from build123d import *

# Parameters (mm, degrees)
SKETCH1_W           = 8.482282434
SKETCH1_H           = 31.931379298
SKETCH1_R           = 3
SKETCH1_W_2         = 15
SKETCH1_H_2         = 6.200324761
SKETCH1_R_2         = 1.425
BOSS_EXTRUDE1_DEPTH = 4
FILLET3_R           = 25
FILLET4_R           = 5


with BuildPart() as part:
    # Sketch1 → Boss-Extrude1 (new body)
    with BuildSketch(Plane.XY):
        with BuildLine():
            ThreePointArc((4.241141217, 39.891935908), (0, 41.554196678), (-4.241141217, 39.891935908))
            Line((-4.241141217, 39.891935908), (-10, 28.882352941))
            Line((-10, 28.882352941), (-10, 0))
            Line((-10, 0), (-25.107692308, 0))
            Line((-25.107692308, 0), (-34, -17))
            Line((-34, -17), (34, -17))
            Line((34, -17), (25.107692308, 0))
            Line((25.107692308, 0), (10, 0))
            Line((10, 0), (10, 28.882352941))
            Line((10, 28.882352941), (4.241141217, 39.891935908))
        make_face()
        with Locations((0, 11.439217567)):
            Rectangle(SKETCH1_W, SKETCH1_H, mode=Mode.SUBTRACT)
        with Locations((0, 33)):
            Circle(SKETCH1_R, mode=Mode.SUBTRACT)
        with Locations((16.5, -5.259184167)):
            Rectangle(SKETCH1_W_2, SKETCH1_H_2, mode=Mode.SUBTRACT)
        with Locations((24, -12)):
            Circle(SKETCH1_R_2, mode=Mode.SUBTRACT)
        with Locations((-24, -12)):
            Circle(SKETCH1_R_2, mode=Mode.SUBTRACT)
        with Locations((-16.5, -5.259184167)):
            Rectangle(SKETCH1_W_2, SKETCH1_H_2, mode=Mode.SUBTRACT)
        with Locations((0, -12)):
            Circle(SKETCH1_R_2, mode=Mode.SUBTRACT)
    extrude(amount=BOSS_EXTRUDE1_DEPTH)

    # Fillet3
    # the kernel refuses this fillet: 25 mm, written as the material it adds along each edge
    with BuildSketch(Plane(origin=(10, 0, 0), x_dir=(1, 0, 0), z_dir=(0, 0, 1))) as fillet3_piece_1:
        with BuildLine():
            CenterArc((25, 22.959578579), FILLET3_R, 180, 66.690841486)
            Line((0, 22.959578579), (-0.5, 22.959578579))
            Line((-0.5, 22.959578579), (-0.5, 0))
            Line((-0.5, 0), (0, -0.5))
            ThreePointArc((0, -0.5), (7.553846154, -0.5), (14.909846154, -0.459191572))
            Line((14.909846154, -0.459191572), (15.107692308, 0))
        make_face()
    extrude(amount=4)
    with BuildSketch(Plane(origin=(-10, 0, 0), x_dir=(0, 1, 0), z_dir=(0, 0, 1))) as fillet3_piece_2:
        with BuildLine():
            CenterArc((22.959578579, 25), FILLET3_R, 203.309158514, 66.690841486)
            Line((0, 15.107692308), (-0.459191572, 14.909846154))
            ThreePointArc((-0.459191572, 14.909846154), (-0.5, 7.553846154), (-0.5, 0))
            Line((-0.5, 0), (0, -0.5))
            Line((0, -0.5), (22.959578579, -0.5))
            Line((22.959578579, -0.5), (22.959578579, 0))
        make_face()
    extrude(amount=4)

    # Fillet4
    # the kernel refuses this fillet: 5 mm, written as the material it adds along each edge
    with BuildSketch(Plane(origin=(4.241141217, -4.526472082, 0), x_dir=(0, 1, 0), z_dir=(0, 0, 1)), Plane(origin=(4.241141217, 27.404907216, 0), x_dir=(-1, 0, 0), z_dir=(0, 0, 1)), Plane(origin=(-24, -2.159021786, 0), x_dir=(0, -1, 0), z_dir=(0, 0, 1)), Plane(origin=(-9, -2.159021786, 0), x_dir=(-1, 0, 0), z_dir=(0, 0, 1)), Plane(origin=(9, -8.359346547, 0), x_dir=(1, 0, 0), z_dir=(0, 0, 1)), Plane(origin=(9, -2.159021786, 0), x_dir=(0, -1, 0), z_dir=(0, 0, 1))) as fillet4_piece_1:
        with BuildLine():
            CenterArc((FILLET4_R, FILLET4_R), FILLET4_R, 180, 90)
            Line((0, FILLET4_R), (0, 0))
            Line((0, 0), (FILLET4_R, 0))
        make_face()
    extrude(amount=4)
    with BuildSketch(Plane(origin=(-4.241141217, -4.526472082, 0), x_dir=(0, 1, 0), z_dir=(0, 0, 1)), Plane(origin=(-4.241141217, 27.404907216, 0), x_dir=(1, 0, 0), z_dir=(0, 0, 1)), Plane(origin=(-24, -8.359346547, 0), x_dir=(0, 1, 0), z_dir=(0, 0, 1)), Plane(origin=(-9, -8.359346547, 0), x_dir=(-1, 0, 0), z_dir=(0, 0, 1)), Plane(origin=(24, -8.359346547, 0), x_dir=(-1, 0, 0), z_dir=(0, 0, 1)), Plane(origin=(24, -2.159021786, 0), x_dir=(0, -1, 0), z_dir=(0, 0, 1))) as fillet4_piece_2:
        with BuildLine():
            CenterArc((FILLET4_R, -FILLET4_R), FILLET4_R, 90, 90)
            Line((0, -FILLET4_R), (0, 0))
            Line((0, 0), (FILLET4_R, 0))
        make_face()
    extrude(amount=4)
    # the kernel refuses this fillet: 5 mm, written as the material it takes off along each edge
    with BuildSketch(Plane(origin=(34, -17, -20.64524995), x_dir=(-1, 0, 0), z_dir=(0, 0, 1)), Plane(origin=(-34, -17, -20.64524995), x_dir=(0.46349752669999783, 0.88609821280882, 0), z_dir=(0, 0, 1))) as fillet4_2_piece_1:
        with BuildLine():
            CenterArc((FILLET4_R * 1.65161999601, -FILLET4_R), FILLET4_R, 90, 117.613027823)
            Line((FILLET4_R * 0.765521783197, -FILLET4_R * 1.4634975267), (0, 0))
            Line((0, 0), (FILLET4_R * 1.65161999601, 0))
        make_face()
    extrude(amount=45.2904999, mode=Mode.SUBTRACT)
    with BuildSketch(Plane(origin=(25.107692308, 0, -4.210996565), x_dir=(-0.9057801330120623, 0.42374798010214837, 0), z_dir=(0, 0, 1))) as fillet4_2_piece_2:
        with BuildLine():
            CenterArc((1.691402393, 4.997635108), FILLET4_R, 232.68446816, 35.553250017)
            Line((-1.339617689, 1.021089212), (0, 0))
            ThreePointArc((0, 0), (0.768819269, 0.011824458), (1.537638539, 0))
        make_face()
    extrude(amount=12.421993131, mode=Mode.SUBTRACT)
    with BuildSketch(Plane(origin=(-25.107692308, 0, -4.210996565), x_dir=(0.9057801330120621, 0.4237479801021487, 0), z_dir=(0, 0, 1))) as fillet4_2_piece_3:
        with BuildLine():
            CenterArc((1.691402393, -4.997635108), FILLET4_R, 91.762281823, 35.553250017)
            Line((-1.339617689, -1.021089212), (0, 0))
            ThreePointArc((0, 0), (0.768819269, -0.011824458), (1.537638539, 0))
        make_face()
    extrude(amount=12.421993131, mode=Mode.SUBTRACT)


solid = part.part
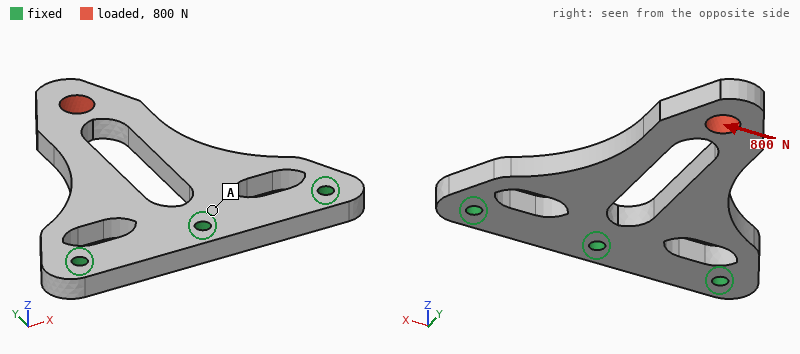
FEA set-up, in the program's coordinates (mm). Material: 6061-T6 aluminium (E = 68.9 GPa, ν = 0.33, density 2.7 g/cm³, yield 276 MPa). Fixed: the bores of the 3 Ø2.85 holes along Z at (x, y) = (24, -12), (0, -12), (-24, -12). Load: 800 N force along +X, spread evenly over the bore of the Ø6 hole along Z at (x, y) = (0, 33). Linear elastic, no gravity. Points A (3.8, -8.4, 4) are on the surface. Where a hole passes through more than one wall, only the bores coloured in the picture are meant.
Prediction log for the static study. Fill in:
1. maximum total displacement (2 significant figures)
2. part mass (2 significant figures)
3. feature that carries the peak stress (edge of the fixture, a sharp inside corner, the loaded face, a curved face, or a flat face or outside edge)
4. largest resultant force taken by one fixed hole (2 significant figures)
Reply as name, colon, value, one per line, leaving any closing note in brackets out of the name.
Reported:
maximum total displacement: 0.11 mm
part mass: 16 g
feature that carries the peak stress: a curved face
largest resultant force taken by one fixed hole: 780 N
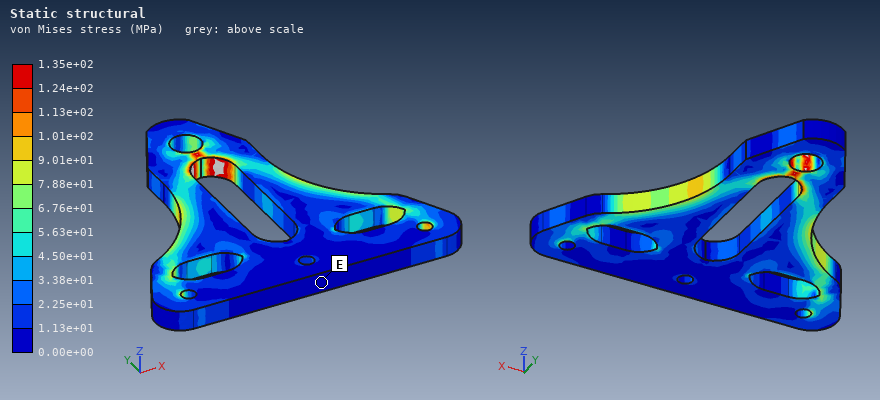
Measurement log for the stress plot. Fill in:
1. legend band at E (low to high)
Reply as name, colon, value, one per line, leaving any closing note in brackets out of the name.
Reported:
legend band at E: 0.00e+00 to 1.13e+01 MPa
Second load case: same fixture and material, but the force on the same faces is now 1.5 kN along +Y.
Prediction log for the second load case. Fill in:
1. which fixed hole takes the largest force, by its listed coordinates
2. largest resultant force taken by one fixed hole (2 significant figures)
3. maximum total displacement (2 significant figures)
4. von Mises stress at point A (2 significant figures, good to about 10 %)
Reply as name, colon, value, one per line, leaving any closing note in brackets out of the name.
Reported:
which fixed hole takes the largest force, by its listed coordinates: (0, -12)
largest resultant force taken by one fixed hole: 890 N
maximum total displacement: 21 µm
von Mises stress at point A: 19 MPa
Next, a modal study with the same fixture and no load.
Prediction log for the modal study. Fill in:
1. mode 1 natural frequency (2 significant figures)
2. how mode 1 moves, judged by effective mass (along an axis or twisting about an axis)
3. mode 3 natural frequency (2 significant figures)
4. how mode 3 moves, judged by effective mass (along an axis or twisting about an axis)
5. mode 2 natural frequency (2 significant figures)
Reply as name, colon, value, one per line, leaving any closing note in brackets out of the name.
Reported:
mode 1 natural frequency: 1500 Hz
how mode 1 moves, judged by effective mass: along Z
mode 3 natural frequency: 7300 Hz
how mode 3 moves, judged by effective mass: along Z
mode 2 natural frequency: 6000 Hz
